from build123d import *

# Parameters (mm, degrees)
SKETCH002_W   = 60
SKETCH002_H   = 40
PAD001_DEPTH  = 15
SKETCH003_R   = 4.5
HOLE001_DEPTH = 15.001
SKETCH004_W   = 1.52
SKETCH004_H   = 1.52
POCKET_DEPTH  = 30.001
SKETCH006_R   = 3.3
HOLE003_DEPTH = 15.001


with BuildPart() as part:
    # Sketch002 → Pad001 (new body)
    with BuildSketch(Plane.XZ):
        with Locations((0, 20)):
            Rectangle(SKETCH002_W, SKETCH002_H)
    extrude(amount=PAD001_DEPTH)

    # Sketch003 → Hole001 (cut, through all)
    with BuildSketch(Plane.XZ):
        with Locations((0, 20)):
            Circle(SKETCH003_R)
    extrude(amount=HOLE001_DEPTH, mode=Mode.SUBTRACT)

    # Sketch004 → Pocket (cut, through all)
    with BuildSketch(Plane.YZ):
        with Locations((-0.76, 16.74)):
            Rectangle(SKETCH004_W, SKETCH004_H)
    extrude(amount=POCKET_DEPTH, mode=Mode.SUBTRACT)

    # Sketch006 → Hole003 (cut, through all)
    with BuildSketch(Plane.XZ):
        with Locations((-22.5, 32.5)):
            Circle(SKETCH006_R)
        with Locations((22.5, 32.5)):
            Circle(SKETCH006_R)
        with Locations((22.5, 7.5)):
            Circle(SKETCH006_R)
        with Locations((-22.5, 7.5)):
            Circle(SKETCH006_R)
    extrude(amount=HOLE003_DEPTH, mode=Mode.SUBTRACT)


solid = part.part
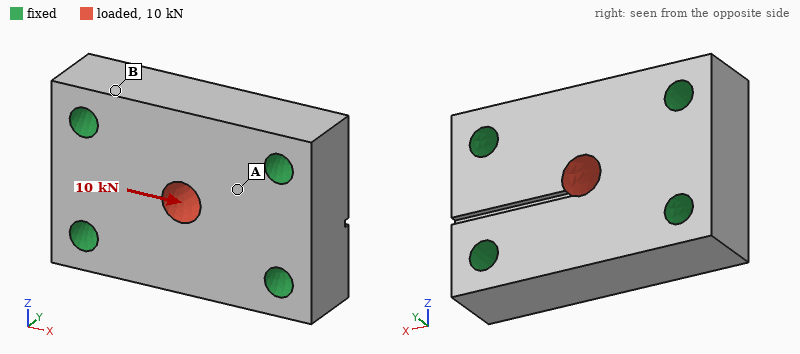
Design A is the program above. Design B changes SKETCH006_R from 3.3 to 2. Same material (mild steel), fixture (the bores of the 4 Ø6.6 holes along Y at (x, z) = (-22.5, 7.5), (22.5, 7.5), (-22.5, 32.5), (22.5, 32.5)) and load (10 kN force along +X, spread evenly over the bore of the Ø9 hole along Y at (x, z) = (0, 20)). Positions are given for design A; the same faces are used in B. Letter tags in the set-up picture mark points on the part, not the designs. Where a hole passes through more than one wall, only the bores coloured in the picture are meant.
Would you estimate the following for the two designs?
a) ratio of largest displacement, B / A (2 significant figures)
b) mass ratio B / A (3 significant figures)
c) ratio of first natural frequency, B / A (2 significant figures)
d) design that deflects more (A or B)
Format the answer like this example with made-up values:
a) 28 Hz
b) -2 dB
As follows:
a) 1.1
b) 1.04
c) 0.87
d) B
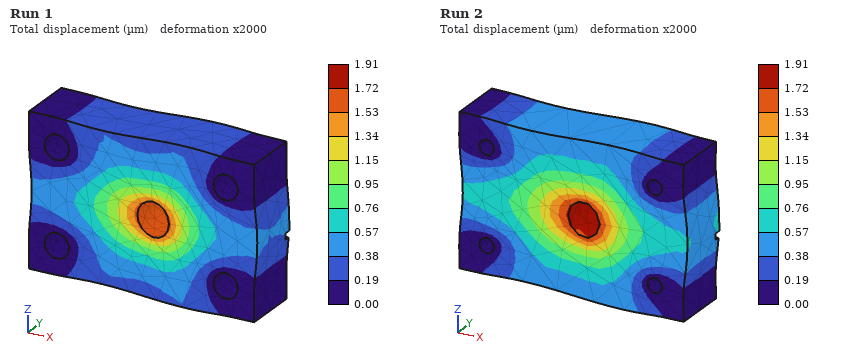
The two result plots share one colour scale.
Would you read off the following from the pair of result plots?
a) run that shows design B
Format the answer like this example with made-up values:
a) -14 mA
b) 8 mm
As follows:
a) Run 2
